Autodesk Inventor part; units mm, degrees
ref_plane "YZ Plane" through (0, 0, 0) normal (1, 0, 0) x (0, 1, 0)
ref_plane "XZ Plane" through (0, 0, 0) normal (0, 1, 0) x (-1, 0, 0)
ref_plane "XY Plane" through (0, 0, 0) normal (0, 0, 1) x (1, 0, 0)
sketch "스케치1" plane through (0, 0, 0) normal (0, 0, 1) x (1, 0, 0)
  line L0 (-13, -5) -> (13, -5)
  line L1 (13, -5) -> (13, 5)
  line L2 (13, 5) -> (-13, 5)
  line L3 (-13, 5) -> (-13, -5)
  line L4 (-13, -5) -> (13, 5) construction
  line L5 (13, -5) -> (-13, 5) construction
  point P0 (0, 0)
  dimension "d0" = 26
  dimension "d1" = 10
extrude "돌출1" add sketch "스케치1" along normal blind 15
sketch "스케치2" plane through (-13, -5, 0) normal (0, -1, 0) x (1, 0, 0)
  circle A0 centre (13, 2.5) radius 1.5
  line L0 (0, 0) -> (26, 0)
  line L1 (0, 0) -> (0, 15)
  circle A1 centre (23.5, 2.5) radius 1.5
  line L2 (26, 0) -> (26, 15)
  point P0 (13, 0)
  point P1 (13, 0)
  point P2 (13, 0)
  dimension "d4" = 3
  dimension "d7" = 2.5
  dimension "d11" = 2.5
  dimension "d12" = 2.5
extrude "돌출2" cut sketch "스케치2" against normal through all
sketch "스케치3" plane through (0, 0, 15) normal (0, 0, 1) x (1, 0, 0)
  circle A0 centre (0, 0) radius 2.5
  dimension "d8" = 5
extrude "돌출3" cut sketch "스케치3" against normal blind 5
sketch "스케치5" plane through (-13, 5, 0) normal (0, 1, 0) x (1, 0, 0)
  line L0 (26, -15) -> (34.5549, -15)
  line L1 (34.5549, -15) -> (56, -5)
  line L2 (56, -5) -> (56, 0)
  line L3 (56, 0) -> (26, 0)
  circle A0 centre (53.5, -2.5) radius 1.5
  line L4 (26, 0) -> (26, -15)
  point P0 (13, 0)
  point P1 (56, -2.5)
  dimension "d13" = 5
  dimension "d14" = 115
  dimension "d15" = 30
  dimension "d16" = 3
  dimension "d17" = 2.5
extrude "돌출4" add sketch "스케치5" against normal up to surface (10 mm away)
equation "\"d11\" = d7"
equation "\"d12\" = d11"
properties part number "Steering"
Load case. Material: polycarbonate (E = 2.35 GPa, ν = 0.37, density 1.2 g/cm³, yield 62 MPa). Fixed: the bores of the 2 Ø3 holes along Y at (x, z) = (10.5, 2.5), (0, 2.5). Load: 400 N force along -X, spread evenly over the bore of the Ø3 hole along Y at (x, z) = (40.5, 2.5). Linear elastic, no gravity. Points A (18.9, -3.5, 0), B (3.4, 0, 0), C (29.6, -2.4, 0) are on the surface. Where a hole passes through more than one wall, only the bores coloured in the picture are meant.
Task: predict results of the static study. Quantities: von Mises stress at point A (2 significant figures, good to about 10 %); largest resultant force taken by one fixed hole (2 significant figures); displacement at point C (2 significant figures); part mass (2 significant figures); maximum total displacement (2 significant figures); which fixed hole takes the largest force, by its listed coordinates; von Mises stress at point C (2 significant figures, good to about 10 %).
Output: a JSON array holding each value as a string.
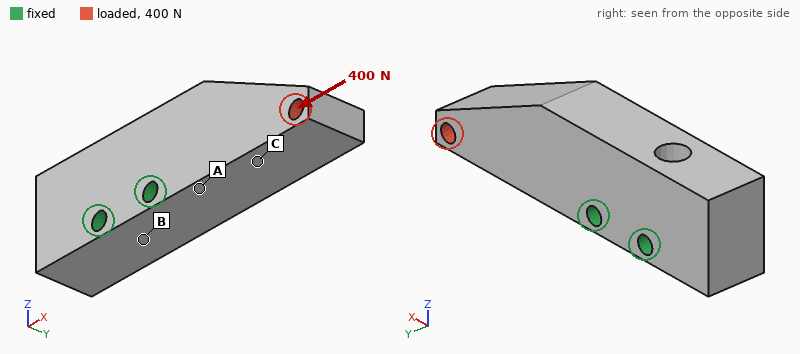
["8.2 MPa", "380 N", "0.085 mm", "8.4 g", "0.22 mm", "(10.5, 2.5)", "9.6 MPa"]
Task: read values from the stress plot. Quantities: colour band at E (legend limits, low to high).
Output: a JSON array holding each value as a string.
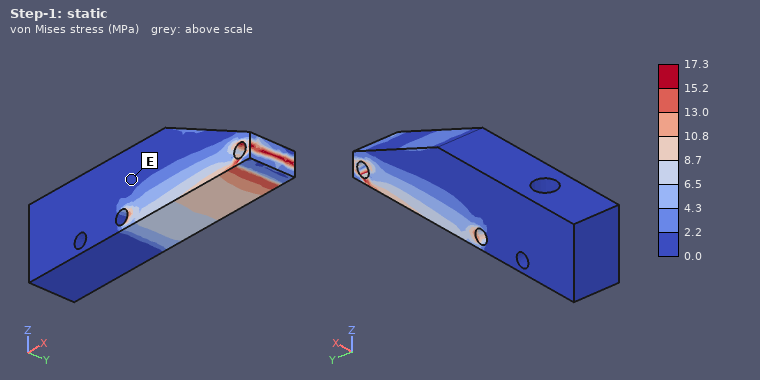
["0.0 to 2.2 MPa"]
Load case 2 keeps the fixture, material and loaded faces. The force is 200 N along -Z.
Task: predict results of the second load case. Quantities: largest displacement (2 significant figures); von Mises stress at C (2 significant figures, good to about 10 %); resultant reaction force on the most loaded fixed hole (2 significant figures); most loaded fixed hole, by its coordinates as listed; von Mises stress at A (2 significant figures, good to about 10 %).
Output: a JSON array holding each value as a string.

["0.70 mm", "11 MPa", "660 N", "(10.5, 2.5)", "12 MPa"]
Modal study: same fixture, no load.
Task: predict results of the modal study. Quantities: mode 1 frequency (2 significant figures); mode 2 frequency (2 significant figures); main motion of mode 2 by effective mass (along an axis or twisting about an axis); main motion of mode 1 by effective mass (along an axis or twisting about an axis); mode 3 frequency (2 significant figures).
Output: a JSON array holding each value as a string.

["2500 Hz", "2900 Hz", "along Z", "along Y", "6400 Hz"]
